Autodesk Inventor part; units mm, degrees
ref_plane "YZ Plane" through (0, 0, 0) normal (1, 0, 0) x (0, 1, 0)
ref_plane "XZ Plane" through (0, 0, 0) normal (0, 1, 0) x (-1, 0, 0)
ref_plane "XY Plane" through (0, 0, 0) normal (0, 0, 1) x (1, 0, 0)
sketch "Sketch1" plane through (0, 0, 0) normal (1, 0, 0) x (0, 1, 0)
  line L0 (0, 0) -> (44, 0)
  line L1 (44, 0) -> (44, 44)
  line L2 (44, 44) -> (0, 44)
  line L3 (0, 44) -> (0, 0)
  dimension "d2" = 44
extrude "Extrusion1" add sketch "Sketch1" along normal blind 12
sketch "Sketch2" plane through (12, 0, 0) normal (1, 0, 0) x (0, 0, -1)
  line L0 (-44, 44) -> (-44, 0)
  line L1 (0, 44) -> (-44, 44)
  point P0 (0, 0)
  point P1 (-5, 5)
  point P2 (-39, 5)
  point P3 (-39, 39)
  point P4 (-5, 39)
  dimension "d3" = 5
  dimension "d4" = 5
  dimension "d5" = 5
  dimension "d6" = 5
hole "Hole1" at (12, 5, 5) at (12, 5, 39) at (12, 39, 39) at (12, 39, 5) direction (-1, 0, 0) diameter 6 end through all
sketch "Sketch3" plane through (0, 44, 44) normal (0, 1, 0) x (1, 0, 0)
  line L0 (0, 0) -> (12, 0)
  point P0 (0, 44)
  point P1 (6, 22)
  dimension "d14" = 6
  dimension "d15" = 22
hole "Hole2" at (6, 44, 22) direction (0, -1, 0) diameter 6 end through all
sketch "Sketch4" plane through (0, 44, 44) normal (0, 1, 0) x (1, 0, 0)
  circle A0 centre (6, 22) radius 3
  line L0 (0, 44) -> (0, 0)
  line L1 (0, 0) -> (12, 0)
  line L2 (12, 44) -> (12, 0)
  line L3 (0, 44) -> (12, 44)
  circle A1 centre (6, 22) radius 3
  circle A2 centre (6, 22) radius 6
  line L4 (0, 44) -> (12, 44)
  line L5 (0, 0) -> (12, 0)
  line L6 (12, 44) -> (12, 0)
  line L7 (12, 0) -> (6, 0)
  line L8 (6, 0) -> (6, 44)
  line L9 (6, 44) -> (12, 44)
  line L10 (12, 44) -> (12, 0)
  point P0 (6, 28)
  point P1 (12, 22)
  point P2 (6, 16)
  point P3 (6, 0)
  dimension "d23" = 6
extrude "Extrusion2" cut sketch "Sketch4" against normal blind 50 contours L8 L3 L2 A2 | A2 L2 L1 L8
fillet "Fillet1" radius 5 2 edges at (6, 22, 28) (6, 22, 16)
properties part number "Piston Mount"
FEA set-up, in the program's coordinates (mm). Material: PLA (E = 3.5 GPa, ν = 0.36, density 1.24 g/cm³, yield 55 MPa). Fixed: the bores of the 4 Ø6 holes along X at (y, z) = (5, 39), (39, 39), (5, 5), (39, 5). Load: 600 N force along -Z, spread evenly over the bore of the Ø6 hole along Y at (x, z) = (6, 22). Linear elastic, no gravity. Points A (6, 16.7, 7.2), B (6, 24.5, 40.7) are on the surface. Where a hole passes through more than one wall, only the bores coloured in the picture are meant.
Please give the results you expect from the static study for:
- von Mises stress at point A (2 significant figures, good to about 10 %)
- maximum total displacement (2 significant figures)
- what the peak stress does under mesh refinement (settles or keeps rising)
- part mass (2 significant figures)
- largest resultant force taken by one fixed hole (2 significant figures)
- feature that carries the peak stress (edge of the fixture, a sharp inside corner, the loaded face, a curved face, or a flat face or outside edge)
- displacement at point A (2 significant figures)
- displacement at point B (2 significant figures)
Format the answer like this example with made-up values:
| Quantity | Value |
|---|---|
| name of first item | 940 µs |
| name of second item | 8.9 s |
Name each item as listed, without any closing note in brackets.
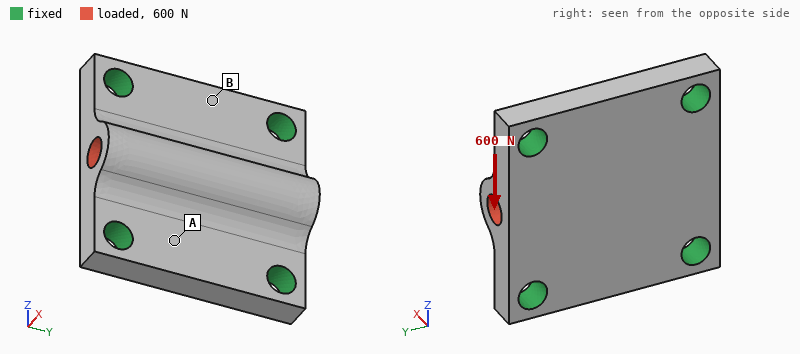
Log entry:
| Quantity | Value |
|---|---|
| von Mises stress at point A | 0.87 MPa |
| maximum total displacement | 14 µm |
| what the peak stress does under mesh refinement | keeps rising |
| part mass | 15 g |
| largest resultant force taken by one fixed hole | 160 N |
| feature that carries the peak stress | edge of the fixture |
| displacement at point A | 6.9 µm |
| displacement at point B | 7.5 µm |
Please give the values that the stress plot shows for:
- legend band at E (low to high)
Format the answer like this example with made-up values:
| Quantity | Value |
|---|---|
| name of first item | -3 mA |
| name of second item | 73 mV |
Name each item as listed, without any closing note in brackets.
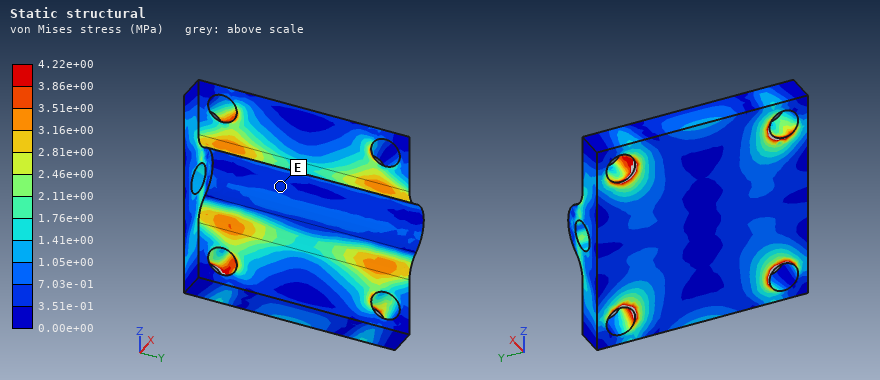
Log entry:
| Quantity | Value |
|---|---|
| legend band at E | 3.51e-01 to 7.03e-01 MPa |
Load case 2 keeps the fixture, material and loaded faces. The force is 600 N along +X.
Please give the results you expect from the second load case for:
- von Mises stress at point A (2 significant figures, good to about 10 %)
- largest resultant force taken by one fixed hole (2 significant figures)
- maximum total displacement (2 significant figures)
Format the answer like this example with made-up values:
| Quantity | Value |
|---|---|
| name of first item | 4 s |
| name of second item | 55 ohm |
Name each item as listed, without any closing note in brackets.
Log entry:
| Quantity | Value |
|---|---|
| von Mises stress at point A | 1.3 MPa |
| largest resultant force taken by one fixed hole | 150 N |
| maximum total displacement | 51 µm |
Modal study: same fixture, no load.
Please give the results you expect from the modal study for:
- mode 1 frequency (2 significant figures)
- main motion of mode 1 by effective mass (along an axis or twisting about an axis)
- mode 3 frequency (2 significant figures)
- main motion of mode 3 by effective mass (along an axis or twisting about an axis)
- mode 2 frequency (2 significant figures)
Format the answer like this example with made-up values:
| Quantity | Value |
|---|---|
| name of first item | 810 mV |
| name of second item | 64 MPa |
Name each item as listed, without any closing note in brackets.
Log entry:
| Quantity | Value |
|---|---|
| mode 1 frequency | 6600 Hz |
| main motion of mode 1 by effective mass | along X |
| mode 3 frequency | 10000 Hz |
| main motion of mode 3 by effective mass | twisting about Y |
| mode 2 frequency | 9300 Hz |
